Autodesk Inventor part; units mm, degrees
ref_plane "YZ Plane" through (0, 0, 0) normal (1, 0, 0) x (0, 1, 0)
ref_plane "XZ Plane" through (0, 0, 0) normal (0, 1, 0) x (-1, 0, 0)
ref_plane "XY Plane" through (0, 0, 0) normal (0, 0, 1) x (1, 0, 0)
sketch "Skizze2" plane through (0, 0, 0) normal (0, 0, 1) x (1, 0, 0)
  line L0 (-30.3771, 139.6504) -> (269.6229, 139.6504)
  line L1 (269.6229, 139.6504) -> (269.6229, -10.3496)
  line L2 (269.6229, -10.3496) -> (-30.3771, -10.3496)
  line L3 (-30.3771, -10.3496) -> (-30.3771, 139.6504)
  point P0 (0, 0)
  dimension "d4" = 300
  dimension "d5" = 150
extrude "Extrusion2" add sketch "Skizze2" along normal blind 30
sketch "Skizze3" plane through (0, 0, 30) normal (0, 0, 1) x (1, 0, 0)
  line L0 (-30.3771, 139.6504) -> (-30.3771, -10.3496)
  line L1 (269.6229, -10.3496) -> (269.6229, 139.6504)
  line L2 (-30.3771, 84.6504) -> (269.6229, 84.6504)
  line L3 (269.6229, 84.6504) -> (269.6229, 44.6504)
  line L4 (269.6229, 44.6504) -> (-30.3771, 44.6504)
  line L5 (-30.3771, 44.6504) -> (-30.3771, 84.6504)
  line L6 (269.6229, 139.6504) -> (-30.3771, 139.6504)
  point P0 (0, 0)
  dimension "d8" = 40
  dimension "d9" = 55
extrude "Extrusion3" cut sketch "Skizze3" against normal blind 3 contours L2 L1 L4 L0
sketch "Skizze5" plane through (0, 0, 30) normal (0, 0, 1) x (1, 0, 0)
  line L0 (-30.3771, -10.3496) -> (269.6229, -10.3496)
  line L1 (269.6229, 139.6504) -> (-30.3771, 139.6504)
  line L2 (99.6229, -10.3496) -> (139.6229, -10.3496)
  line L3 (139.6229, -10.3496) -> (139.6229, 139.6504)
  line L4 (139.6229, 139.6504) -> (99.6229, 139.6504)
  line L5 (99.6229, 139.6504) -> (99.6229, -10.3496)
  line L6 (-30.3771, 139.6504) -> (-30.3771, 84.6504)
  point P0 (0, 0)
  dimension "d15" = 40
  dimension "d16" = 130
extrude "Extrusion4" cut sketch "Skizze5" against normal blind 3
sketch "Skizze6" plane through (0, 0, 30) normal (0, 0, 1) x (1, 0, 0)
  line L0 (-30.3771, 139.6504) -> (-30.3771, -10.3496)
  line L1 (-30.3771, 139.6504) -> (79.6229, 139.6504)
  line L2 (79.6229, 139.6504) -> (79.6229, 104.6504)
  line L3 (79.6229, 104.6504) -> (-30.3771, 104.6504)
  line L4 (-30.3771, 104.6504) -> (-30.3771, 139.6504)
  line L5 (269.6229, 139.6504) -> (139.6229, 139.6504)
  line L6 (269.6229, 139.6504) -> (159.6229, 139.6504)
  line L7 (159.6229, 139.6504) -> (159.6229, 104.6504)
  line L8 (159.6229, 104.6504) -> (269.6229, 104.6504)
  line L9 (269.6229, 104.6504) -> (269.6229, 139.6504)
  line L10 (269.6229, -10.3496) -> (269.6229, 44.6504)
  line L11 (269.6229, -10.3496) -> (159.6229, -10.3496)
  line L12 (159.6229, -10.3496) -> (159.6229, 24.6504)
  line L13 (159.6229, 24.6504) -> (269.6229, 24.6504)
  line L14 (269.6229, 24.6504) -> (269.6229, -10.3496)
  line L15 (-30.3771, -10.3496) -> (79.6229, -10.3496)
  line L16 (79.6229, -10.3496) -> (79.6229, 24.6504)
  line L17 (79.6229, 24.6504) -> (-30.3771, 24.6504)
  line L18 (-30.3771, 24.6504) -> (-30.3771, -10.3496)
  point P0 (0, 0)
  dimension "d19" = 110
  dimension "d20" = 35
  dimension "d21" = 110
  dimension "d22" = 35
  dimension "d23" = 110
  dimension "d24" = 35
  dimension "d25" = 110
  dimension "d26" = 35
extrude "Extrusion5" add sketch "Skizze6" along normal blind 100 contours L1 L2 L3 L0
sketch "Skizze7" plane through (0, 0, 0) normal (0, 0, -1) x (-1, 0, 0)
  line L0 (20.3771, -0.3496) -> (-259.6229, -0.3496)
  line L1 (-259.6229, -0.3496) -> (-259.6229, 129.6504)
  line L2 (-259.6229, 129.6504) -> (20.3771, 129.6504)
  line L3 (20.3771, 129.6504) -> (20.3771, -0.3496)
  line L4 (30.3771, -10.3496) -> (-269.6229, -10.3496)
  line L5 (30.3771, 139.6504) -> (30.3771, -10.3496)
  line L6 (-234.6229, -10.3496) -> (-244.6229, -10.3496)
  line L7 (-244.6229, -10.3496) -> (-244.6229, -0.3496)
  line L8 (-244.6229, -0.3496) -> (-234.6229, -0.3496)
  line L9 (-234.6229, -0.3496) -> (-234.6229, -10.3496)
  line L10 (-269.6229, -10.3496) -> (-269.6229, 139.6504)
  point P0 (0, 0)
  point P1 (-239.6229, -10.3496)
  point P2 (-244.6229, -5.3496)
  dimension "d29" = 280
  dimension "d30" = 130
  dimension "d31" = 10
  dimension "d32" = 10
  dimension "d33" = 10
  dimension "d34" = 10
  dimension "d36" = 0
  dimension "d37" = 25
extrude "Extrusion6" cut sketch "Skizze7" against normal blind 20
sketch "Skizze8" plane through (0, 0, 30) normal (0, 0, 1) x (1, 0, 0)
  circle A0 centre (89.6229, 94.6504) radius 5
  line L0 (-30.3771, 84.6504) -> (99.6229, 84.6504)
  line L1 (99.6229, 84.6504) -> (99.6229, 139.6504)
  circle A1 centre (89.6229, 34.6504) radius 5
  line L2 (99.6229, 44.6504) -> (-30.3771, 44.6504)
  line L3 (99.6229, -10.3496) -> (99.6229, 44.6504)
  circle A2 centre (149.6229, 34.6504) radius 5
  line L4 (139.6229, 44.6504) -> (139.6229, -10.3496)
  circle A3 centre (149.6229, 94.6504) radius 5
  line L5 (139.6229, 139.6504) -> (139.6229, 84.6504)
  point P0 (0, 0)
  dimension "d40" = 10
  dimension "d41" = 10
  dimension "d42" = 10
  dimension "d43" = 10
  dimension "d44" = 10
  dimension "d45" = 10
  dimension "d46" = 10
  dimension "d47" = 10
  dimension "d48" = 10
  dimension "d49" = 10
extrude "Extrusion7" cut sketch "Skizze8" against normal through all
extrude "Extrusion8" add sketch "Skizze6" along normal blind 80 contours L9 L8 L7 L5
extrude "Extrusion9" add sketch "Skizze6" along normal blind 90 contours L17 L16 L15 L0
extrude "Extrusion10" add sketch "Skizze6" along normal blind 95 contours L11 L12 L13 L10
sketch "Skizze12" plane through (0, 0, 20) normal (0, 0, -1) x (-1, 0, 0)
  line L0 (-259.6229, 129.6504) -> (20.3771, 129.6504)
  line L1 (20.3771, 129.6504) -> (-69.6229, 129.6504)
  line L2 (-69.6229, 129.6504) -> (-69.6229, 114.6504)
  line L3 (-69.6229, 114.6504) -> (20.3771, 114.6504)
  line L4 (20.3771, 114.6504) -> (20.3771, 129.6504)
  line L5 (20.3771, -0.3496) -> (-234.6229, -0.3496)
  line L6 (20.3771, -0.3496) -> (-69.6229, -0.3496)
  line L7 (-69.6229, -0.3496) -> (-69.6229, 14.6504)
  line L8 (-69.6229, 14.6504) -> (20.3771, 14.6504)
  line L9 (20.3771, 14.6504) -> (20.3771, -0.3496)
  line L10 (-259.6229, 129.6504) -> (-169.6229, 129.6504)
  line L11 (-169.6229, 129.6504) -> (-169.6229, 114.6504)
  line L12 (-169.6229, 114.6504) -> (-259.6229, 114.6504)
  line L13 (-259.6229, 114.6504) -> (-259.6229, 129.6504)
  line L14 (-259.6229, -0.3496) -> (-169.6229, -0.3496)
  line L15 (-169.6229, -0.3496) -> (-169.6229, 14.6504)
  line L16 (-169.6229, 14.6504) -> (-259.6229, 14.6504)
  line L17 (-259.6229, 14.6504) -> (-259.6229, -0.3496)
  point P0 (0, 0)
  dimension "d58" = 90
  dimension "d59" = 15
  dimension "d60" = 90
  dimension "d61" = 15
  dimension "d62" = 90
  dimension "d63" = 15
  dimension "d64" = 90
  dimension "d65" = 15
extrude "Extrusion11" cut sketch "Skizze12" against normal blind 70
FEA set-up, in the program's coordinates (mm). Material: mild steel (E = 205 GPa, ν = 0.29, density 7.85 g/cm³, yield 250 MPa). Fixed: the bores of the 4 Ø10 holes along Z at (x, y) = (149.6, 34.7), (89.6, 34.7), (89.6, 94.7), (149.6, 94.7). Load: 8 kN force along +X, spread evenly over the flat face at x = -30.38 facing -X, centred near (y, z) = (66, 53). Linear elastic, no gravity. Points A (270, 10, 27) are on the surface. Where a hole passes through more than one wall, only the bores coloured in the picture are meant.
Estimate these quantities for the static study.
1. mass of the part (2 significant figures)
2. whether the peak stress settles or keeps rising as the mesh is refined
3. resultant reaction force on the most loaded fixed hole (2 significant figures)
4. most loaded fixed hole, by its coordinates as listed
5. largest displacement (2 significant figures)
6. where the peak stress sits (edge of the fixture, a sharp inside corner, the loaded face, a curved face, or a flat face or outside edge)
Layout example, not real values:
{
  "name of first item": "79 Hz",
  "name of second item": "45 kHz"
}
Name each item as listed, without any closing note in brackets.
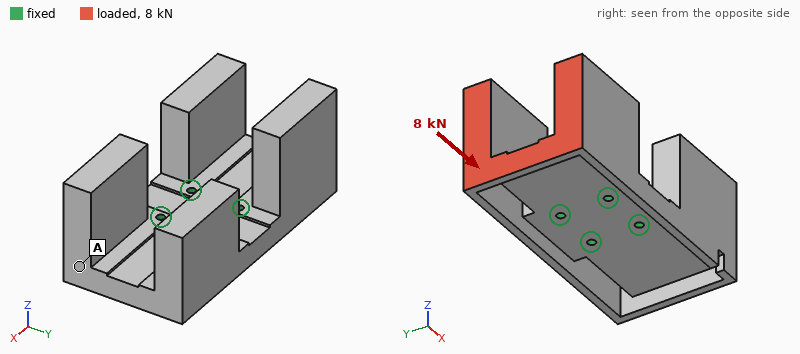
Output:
{
  "mass of the part": "13 kg",
  "whether the peak stress settles or keeps rising as the mesh is refined": "keeps rising",
  "resultant reaction force on the most loaded fixed hole": "4.1 kN",
  "most loaded fixed hole, by its coordinates as listed": "(89.6, 94.7)",
  "largest displacement": "0.17 mm",
  "where the peak stress sits": "edge of the fixture"
}
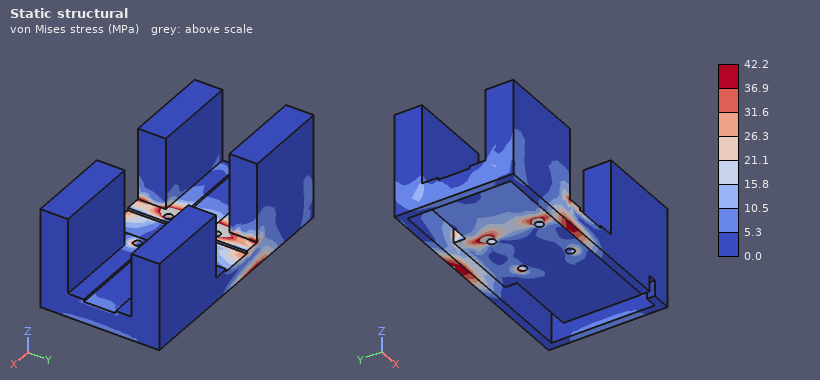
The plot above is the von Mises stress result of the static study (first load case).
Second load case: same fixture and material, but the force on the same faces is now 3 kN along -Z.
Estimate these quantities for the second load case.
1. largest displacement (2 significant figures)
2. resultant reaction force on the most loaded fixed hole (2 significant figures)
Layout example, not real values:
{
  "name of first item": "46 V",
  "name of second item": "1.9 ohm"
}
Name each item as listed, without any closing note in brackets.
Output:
{
  "largest displacement": "0.25 mm",
  "resultant reaction force on the most loaded fixed hole": "3.6 kN"
}
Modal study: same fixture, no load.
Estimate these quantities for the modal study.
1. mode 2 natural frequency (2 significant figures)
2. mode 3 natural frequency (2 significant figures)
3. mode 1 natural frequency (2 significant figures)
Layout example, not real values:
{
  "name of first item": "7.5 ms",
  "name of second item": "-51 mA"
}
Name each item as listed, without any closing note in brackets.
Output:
{
  "mode 2 natural frequency": "340 Hz",
  "mode 3 natural frequency": "370 Hz",
  "mode 1 natural frequency": "310 Hz"
}
